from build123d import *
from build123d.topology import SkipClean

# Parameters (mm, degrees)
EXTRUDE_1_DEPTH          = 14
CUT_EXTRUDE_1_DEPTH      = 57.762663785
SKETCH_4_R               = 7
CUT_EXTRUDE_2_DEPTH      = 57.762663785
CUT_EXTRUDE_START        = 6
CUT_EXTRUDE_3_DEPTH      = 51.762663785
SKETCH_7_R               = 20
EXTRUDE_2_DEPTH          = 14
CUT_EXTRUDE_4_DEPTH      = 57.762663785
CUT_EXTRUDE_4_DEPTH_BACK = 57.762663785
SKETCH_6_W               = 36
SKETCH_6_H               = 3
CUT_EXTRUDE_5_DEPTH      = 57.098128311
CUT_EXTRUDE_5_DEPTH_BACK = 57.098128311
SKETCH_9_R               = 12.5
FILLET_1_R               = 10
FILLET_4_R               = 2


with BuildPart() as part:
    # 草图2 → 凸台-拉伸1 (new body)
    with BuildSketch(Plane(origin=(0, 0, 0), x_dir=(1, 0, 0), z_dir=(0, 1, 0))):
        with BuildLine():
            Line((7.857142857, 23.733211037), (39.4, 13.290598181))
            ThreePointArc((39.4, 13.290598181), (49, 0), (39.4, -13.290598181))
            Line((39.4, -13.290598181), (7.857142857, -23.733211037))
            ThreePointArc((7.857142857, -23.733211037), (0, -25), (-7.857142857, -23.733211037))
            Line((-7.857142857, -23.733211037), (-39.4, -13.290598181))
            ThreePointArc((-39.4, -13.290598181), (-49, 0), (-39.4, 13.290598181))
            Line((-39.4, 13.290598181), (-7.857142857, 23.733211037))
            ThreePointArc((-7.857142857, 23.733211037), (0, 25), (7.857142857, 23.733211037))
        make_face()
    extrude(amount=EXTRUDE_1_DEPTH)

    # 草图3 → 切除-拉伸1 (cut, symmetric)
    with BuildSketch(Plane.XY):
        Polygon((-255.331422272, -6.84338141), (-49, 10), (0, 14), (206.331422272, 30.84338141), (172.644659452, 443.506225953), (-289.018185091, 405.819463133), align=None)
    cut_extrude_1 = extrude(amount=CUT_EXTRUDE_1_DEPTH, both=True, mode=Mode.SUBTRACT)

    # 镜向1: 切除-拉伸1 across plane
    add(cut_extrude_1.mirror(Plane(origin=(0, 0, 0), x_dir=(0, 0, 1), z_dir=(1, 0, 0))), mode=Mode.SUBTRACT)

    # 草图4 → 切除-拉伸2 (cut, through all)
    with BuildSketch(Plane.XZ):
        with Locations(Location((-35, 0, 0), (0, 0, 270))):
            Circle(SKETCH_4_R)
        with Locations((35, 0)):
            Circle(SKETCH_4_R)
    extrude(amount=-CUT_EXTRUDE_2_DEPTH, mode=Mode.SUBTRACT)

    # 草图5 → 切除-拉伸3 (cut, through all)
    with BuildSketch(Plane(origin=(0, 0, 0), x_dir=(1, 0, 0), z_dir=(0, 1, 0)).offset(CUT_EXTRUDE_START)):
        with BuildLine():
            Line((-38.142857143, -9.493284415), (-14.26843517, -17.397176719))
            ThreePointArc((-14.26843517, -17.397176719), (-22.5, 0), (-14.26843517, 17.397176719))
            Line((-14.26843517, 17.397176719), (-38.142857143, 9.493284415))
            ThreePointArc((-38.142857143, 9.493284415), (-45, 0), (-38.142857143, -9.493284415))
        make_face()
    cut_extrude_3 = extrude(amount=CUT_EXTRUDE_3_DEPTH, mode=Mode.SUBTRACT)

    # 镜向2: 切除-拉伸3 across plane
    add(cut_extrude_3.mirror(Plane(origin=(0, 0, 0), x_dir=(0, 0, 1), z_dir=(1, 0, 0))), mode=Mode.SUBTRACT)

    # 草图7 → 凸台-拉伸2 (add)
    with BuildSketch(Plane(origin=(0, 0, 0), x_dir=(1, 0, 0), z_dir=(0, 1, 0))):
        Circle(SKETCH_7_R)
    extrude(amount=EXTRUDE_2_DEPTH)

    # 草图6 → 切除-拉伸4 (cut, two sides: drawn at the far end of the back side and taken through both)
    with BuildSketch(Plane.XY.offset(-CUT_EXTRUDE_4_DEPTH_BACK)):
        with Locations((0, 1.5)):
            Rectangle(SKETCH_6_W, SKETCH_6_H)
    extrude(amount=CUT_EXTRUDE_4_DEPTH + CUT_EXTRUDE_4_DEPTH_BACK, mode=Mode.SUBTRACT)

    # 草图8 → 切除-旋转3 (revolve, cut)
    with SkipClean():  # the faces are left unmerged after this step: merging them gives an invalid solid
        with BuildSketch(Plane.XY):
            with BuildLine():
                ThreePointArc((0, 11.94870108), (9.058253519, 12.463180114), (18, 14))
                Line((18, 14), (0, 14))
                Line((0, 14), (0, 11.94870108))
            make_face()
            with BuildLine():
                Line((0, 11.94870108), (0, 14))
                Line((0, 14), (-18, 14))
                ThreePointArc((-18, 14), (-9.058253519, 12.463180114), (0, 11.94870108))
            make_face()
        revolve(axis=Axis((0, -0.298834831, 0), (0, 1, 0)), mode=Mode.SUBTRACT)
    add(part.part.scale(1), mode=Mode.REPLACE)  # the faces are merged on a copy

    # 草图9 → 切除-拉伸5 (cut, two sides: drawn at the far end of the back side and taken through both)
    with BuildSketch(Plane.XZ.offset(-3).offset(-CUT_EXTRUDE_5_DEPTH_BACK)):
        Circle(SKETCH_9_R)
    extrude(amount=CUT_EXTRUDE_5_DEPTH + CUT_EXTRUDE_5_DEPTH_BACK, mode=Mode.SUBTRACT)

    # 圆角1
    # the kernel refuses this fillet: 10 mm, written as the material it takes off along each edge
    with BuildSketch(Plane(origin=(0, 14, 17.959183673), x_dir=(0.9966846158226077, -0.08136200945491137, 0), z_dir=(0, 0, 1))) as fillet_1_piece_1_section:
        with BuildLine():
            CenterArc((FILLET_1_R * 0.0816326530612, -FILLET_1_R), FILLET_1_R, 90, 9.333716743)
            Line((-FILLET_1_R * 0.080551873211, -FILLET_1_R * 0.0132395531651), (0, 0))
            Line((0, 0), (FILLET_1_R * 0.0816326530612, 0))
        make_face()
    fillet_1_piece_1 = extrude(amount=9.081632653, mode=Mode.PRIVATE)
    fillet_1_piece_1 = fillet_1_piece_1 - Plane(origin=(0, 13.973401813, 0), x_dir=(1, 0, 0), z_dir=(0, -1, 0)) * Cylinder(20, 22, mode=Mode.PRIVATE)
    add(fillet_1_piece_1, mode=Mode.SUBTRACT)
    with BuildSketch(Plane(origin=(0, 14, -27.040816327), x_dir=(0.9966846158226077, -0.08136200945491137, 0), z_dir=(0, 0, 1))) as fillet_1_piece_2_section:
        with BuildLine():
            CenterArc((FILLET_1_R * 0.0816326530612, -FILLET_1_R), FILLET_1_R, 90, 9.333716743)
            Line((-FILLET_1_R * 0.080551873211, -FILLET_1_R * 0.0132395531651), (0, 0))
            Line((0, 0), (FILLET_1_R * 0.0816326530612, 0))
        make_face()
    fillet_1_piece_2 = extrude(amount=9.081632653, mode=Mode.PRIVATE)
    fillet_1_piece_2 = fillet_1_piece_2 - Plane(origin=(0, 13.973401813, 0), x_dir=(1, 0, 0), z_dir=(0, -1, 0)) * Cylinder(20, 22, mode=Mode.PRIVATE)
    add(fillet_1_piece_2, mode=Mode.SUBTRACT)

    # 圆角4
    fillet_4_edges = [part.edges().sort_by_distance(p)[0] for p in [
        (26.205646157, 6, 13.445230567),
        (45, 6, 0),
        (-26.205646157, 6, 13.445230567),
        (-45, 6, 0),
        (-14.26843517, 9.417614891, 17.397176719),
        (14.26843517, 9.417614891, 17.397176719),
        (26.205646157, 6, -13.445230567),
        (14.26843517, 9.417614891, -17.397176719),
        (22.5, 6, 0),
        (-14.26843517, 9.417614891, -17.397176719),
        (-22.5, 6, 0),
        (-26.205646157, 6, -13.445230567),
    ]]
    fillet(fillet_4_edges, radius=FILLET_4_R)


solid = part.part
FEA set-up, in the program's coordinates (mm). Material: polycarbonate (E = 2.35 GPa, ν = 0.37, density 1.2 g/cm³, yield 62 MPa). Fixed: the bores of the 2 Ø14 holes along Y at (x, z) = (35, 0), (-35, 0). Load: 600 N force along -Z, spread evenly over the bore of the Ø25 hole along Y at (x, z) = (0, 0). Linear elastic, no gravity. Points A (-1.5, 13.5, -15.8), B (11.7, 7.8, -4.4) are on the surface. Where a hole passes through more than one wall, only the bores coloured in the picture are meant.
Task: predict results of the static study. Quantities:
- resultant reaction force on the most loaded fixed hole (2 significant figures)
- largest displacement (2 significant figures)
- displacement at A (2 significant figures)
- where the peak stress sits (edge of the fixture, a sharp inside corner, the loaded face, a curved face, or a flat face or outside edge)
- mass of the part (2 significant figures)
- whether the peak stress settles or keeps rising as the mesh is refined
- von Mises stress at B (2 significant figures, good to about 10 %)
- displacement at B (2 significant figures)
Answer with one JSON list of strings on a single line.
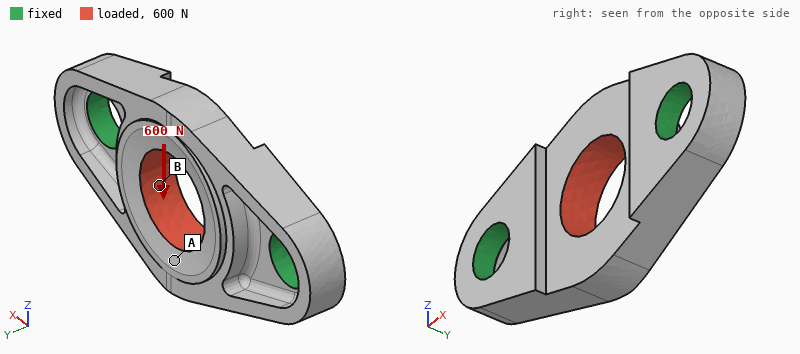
["300 N", "0.15 mm", "0.12 mm", "edge of the fixture", "31 g", "keeps rising", "1.9 MPa", "0.062 mm"]
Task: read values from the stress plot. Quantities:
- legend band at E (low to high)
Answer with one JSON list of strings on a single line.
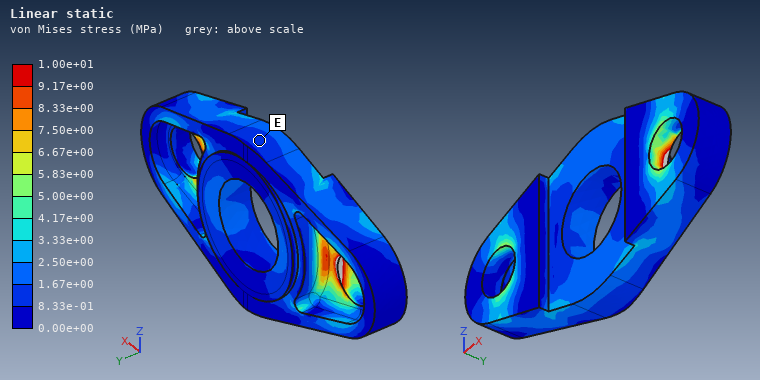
["8.33e-01 to 1.67e+00 MPa"]
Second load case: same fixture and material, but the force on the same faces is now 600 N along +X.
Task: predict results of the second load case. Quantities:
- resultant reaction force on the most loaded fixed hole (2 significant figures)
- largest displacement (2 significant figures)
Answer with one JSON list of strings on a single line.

["300 N", "25 µm"]
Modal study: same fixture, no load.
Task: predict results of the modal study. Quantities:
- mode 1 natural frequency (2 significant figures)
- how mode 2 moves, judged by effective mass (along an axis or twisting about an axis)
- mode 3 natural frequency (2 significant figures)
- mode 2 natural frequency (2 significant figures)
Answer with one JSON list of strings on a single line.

["1900 Hz", "along Y", "4900 Hz", "2500 Hz"]
